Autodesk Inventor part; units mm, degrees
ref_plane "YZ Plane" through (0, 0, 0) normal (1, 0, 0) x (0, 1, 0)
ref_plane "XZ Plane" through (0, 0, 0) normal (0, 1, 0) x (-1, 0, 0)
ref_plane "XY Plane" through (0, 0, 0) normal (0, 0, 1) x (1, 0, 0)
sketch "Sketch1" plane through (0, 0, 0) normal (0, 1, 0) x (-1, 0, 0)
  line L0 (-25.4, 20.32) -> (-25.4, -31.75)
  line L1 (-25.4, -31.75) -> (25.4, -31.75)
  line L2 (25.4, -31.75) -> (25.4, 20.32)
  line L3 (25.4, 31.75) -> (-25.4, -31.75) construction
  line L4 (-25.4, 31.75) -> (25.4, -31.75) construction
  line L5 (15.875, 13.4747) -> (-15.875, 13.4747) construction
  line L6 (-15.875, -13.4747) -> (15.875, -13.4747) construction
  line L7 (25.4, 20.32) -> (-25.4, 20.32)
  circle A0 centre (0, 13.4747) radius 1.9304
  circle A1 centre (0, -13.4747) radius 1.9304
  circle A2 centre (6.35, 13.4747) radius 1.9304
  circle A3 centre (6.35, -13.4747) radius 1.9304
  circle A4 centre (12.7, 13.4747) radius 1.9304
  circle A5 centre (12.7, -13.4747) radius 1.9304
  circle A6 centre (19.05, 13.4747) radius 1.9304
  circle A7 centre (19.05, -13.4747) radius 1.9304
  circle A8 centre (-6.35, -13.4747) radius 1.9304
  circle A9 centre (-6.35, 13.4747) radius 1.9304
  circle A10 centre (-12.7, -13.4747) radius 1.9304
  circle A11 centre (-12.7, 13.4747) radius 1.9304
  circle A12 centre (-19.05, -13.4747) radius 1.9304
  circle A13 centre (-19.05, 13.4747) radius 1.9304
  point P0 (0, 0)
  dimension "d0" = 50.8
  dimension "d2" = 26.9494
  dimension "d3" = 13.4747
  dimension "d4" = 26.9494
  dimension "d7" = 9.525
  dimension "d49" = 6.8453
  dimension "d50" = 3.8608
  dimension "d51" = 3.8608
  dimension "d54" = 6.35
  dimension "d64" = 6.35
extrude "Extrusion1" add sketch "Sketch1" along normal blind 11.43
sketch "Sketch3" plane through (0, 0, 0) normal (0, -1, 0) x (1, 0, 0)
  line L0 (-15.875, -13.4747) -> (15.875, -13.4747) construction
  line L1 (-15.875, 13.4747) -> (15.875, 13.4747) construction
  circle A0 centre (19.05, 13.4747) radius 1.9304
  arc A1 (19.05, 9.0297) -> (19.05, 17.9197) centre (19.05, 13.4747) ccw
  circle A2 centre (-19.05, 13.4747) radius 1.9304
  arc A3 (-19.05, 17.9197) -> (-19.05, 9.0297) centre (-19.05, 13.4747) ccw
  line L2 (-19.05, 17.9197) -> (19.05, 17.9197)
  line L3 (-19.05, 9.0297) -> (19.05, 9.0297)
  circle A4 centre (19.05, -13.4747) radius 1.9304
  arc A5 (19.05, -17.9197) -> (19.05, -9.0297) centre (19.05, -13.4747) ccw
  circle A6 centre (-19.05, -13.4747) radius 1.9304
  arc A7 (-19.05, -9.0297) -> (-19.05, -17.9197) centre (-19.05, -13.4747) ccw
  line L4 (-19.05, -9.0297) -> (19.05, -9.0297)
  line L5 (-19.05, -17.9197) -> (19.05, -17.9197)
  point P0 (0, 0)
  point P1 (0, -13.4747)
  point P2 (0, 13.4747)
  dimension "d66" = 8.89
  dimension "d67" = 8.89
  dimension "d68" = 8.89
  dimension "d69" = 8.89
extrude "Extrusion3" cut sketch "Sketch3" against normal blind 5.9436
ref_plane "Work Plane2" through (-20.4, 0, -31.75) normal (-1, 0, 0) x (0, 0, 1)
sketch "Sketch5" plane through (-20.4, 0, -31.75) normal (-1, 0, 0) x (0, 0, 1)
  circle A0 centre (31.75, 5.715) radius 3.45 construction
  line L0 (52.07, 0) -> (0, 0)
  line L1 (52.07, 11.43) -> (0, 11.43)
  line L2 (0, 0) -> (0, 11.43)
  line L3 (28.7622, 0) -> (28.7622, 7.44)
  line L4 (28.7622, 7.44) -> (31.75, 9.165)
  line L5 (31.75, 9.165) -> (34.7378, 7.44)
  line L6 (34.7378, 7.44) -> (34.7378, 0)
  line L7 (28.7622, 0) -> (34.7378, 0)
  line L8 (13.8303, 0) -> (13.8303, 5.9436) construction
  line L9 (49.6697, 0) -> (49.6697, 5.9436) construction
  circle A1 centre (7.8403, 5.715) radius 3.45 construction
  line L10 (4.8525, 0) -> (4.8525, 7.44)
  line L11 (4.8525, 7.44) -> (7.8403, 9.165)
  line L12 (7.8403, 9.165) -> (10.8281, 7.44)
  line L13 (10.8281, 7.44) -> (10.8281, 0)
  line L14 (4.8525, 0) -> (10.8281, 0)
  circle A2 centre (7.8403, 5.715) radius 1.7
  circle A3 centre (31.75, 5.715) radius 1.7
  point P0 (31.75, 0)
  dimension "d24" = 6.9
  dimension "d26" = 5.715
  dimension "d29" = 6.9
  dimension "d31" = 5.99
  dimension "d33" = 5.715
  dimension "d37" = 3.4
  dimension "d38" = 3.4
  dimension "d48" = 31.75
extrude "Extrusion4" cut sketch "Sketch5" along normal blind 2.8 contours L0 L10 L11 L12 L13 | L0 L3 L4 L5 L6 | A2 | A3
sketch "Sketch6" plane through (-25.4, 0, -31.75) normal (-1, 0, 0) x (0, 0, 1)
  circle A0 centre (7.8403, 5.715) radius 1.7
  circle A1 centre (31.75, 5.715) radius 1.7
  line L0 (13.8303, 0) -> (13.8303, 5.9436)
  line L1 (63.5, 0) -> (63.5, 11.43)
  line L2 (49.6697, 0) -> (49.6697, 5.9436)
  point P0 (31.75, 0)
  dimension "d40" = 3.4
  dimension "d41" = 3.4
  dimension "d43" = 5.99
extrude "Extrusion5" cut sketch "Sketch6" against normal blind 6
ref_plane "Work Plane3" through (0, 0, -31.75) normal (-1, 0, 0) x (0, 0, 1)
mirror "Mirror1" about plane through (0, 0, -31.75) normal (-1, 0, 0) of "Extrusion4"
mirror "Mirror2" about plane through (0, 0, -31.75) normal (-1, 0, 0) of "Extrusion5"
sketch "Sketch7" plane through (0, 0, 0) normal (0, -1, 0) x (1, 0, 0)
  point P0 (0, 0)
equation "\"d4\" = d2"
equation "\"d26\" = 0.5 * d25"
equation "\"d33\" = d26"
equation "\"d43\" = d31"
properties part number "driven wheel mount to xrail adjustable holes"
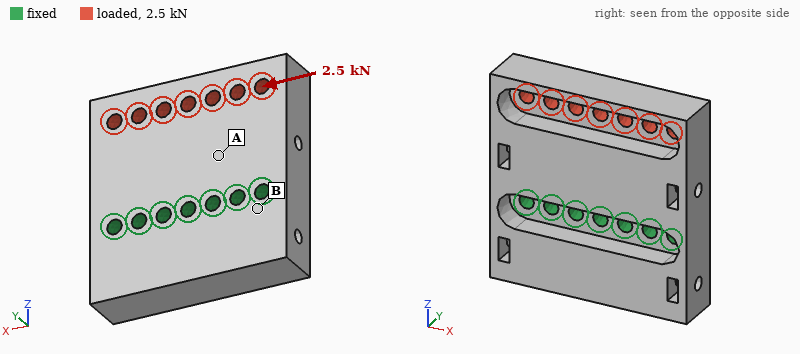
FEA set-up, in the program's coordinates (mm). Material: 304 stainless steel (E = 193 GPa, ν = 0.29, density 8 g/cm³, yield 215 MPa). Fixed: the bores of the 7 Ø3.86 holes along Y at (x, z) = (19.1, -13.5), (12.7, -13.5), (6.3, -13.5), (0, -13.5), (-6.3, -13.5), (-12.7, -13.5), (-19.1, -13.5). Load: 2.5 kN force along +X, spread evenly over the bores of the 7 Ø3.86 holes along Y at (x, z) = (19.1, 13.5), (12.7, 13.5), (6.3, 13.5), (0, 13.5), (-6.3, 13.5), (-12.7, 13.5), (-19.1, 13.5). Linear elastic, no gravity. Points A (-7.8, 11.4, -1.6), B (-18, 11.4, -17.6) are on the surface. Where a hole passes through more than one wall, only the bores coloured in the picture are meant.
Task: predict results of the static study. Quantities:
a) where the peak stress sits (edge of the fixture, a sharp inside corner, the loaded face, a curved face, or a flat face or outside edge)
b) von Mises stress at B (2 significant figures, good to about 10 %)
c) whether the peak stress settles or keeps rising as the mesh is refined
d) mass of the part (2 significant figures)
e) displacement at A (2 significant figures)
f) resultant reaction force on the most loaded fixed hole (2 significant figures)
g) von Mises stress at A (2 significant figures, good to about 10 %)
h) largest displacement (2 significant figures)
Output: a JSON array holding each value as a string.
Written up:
["edge of the fixture", "6.1 MPa", "keeps rising", "190 g", "1.7 µm", "1.3 kN", "20 MPa", "7.0 µm"]
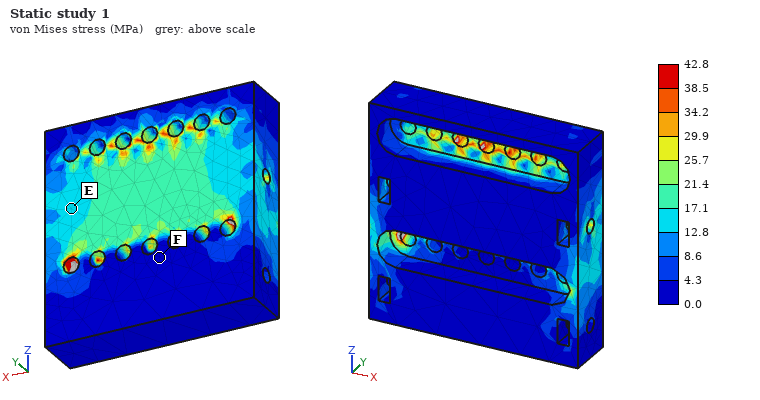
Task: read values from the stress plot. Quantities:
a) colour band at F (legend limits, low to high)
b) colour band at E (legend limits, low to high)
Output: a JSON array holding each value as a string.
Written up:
["0.0 to 4.3 MPa", "12.8 to 17.1 MPa"]
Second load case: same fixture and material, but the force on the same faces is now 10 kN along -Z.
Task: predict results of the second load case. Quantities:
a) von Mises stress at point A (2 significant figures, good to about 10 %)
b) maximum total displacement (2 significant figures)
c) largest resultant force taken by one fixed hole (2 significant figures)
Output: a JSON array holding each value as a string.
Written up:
["46 MPa", "11 µm", "1.8 kN"]
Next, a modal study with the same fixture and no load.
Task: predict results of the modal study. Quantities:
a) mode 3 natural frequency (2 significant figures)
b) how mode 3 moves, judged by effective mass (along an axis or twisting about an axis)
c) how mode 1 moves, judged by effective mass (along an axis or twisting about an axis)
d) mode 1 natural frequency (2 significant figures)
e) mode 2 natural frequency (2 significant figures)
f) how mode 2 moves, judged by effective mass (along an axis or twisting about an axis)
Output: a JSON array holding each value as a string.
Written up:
["11 kHz", "along Y", "along Y", "4700 Hz", "9100 Hz", "twisting about Z"]
